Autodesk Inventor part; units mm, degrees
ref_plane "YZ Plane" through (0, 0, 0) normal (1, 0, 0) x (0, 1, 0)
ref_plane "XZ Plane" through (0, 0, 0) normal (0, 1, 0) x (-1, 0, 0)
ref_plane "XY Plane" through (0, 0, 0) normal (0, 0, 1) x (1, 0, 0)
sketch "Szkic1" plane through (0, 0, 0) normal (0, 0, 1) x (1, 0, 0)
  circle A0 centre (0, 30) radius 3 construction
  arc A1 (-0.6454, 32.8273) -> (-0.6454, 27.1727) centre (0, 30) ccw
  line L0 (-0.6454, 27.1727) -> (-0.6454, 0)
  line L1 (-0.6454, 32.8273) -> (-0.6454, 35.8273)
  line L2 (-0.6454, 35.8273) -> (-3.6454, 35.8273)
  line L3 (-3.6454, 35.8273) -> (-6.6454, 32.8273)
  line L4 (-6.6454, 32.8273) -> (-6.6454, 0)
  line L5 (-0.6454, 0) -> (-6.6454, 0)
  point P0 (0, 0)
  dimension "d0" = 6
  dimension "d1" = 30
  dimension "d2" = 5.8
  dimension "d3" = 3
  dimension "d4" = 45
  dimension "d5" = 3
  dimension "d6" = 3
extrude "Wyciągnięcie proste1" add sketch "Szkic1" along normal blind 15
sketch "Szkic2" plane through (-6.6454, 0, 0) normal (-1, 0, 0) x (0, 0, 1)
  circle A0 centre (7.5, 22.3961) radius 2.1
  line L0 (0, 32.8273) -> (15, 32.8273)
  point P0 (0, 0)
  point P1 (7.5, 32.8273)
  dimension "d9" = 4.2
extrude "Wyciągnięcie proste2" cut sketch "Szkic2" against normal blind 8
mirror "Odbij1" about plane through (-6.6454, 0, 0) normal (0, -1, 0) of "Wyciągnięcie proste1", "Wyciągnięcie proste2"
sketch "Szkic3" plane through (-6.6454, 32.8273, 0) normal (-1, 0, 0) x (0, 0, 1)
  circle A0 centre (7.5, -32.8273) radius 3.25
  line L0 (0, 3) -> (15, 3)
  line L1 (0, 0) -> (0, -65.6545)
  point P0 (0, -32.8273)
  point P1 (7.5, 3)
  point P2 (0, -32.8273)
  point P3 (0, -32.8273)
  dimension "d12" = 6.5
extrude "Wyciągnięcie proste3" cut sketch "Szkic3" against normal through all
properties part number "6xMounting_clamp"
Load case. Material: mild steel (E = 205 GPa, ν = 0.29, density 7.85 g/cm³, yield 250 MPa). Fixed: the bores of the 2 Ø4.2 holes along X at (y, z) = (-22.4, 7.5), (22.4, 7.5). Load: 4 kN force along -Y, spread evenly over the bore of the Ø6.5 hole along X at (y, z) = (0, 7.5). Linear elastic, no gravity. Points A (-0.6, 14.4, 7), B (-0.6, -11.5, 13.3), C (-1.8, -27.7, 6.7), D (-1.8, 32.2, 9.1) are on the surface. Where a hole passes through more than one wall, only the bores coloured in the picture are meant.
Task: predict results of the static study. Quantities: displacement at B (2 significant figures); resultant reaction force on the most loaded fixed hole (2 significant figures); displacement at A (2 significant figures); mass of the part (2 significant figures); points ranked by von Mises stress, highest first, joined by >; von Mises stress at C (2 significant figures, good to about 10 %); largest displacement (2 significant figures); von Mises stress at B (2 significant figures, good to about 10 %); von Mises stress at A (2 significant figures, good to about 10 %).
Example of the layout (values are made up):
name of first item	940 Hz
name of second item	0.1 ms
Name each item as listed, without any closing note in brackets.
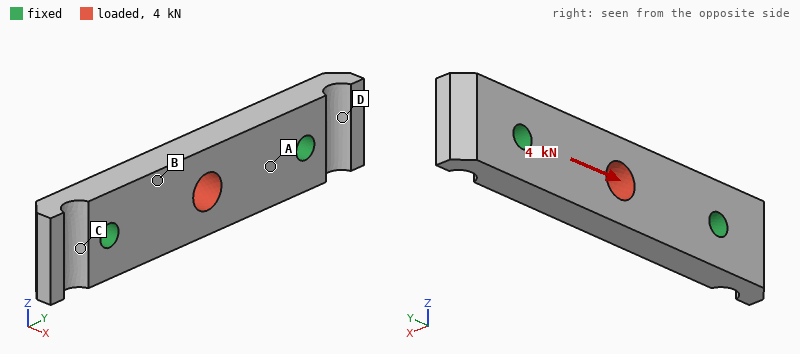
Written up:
displacement at B	1.4 µm
resultant reaction force on the most loaded fixed hole	2.0 kN
displacement at A	0.98 µm
mass of the part	44 g
points ranked by von Mises stress, highest first, joined by >	A > B > C > D
von Mises stress at C	10 MPa
largest displacement	2.8 µm
von Mises stress at B	20 MPa
von Mises stress at A	29 MPa
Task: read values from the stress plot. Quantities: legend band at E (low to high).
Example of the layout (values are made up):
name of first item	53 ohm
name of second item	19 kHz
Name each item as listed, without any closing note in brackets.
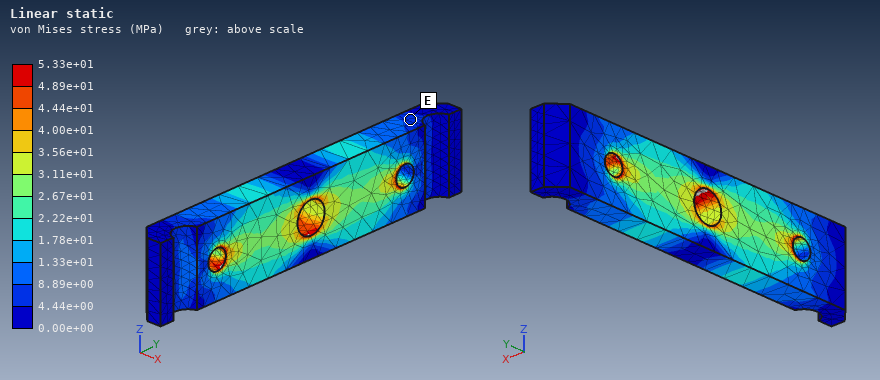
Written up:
legend band at E	4.44e+00 to 8.89e+00 MPa
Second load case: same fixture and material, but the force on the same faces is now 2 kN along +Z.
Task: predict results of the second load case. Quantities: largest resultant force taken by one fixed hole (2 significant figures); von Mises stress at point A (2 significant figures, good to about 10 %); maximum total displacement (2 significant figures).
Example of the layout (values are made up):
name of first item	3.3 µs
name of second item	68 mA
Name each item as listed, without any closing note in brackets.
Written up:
largest resultant force taken by one fixed hole	1.0 kN
von Mises stress at point A	29 MPa
maximum total displacement	8.4 µm
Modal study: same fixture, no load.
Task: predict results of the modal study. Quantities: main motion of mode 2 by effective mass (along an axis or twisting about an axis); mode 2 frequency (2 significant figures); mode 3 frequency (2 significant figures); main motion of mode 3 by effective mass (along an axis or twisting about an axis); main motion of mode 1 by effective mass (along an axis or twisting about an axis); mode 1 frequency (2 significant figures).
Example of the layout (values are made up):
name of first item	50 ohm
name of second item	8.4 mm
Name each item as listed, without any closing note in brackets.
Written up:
main motion of mode 2 by effective mass	along Z
mode 2 frequency	21 kHz
mode 3 frequency	24 kHz
main motion of mode 3 by effective mass	twisting about Y
main motion of mode 1 by effective mass	along X
mode 1 frequency	14 kHz
